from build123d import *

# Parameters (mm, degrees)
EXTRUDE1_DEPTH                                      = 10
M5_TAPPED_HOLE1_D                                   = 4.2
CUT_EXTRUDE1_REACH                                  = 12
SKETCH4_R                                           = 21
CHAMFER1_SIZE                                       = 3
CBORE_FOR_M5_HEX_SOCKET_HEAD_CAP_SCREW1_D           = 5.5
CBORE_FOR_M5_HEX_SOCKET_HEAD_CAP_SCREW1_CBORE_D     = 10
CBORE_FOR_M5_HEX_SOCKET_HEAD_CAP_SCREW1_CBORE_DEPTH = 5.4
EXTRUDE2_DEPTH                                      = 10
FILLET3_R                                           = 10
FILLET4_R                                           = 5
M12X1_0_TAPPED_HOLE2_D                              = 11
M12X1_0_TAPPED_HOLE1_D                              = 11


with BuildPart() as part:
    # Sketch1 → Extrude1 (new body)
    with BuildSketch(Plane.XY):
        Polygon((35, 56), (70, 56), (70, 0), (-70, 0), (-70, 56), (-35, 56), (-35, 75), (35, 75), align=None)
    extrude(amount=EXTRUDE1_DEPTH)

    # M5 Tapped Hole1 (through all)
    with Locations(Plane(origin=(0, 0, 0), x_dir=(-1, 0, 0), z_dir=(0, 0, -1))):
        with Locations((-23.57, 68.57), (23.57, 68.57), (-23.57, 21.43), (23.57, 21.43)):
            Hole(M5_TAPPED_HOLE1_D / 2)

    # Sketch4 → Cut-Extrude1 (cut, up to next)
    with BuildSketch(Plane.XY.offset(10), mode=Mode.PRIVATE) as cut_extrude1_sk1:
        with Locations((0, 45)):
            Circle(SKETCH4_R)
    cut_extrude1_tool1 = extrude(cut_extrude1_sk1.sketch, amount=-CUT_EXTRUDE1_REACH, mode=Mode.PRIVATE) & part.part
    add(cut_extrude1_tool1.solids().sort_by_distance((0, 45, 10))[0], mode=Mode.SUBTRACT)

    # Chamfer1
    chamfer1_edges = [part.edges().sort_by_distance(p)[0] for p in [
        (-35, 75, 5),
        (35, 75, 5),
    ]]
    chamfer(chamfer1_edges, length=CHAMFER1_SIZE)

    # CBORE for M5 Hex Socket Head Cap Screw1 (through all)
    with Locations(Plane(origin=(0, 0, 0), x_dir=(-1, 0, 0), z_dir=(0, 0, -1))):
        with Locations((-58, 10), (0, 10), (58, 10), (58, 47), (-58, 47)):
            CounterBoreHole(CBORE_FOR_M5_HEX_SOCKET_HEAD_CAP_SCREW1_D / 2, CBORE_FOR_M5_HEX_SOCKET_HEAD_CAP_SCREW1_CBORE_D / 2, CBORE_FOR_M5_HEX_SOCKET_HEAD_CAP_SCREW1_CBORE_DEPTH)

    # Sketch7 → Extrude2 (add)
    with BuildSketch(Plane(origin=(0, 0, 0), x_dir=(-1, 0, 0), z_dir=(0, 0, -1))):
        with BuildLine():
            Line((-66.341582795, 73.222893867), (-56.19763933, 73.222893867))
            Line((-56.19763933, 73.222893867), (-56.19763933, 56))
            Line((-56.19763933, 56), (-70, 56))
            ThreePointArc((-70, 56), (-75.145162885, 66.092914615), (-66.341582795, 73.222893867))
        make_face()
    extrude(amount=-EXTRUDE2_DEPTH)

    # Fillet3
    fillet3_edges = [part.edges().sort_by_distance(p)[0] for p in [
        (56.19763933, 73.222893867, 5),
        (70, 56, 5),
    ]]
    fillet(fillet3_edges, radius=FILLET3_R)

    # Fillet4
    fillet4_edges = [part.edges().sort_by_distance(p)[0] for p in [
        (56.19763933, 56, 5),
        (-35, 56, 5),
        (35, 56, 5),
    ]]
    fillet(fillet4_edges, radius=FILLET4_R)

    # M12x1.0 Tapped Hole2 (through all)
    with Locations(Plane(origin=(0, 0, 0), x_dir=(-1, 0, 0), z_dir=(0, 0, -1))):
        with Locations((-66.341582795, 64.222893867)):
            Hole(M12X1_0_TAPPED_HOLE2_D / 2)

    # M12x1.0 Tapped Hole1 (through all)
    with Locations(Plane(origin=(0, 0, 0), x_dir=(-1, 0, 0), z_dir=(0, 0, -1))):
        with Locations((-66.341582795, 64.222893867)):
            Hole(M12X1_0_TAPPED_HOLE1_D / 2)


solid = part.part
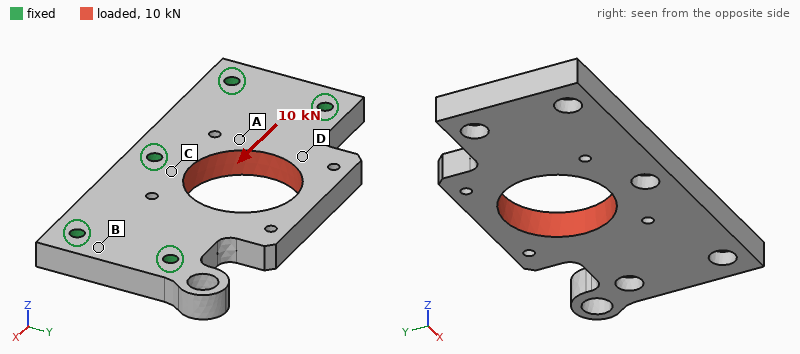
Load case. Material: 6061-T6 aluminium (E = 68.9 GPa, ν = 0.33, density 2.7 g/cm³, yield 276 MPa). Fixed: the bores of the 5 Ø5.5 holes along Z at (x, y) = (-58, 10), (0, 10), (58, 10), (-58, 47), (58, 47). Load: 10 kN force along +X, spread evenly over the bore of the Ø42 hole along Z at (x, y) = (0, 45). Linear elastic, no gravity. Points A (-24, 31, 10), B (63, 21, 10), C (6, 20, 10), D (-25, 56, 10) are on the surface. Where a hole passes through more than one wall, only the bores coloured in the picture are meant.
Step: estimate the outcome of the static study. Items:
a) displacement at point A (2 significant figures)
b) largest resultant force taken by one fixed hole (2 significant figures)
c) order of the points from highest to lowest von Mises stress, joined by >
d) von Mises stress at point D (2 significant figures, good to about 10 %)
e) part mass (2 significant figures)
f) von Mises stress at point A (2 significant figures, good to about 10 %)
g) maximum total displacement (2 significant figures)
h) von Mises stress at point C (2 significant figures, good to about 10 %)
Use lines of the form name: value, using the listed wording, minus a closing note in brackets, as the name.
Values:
displacement at point A: 5.9 µm
largest resultant force taken by one fixed hole: 2.8 kN
order of the points from highest to lowest von Mises stress, joined by >: D > C > A > B
von Mises stress at point D: 24 MPa
part mass: 210 g
von Mises stress at point A: 9.5 MPa
maximum total displacement: 25 µm
von Mises stress at point C: 16 MPa
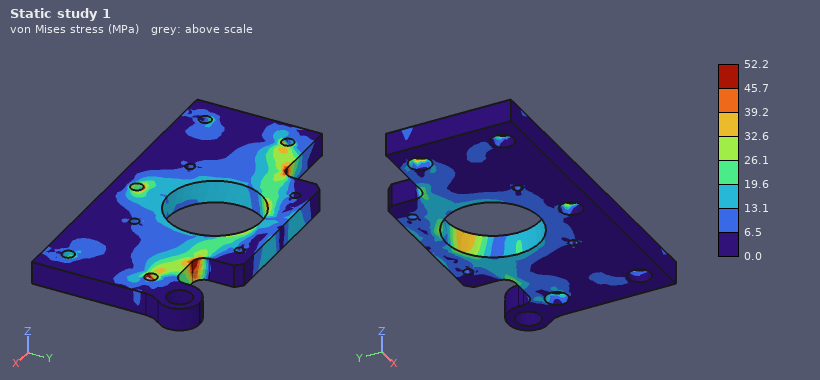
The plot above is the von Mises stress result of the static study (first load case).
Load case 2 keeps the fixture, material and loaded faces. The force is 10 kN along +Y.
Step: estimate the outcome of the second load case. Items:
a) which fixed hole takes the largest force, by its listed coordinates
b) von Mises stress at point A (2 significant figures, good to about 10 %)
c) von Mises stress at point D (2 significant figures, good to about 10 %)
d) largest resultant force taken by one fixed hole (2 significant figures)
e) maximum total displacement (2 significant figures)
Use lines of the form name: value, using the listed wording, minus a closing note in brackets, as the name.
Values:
which fixed hole takes the largest force, by its listed coordinates: (0, 10)
von Mises stress at point A: 12 MPa
von Mises stress at point D: 19 MPa
largest resultant force taken by one fixed hole: 3.9 kN
maximum total displacement: 31 µm
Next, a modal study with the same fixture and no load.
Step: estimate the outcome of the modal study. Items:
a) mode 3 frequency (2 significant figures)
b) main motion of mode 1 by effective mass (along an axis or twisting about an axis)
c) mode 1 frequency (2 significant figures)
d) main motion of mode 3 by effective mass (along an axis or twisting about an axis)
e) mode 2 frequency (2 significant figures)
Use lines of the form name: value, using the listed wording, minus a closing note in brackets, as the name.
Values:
mode 3 frequency: 8700 Hz
main motion of mode 1 by effective mass: along Z
mode 1 frequency: 3000 Hz
main motion of mode 3 by effective mass: along Z
mode 2 frequency: 6200 Hz
